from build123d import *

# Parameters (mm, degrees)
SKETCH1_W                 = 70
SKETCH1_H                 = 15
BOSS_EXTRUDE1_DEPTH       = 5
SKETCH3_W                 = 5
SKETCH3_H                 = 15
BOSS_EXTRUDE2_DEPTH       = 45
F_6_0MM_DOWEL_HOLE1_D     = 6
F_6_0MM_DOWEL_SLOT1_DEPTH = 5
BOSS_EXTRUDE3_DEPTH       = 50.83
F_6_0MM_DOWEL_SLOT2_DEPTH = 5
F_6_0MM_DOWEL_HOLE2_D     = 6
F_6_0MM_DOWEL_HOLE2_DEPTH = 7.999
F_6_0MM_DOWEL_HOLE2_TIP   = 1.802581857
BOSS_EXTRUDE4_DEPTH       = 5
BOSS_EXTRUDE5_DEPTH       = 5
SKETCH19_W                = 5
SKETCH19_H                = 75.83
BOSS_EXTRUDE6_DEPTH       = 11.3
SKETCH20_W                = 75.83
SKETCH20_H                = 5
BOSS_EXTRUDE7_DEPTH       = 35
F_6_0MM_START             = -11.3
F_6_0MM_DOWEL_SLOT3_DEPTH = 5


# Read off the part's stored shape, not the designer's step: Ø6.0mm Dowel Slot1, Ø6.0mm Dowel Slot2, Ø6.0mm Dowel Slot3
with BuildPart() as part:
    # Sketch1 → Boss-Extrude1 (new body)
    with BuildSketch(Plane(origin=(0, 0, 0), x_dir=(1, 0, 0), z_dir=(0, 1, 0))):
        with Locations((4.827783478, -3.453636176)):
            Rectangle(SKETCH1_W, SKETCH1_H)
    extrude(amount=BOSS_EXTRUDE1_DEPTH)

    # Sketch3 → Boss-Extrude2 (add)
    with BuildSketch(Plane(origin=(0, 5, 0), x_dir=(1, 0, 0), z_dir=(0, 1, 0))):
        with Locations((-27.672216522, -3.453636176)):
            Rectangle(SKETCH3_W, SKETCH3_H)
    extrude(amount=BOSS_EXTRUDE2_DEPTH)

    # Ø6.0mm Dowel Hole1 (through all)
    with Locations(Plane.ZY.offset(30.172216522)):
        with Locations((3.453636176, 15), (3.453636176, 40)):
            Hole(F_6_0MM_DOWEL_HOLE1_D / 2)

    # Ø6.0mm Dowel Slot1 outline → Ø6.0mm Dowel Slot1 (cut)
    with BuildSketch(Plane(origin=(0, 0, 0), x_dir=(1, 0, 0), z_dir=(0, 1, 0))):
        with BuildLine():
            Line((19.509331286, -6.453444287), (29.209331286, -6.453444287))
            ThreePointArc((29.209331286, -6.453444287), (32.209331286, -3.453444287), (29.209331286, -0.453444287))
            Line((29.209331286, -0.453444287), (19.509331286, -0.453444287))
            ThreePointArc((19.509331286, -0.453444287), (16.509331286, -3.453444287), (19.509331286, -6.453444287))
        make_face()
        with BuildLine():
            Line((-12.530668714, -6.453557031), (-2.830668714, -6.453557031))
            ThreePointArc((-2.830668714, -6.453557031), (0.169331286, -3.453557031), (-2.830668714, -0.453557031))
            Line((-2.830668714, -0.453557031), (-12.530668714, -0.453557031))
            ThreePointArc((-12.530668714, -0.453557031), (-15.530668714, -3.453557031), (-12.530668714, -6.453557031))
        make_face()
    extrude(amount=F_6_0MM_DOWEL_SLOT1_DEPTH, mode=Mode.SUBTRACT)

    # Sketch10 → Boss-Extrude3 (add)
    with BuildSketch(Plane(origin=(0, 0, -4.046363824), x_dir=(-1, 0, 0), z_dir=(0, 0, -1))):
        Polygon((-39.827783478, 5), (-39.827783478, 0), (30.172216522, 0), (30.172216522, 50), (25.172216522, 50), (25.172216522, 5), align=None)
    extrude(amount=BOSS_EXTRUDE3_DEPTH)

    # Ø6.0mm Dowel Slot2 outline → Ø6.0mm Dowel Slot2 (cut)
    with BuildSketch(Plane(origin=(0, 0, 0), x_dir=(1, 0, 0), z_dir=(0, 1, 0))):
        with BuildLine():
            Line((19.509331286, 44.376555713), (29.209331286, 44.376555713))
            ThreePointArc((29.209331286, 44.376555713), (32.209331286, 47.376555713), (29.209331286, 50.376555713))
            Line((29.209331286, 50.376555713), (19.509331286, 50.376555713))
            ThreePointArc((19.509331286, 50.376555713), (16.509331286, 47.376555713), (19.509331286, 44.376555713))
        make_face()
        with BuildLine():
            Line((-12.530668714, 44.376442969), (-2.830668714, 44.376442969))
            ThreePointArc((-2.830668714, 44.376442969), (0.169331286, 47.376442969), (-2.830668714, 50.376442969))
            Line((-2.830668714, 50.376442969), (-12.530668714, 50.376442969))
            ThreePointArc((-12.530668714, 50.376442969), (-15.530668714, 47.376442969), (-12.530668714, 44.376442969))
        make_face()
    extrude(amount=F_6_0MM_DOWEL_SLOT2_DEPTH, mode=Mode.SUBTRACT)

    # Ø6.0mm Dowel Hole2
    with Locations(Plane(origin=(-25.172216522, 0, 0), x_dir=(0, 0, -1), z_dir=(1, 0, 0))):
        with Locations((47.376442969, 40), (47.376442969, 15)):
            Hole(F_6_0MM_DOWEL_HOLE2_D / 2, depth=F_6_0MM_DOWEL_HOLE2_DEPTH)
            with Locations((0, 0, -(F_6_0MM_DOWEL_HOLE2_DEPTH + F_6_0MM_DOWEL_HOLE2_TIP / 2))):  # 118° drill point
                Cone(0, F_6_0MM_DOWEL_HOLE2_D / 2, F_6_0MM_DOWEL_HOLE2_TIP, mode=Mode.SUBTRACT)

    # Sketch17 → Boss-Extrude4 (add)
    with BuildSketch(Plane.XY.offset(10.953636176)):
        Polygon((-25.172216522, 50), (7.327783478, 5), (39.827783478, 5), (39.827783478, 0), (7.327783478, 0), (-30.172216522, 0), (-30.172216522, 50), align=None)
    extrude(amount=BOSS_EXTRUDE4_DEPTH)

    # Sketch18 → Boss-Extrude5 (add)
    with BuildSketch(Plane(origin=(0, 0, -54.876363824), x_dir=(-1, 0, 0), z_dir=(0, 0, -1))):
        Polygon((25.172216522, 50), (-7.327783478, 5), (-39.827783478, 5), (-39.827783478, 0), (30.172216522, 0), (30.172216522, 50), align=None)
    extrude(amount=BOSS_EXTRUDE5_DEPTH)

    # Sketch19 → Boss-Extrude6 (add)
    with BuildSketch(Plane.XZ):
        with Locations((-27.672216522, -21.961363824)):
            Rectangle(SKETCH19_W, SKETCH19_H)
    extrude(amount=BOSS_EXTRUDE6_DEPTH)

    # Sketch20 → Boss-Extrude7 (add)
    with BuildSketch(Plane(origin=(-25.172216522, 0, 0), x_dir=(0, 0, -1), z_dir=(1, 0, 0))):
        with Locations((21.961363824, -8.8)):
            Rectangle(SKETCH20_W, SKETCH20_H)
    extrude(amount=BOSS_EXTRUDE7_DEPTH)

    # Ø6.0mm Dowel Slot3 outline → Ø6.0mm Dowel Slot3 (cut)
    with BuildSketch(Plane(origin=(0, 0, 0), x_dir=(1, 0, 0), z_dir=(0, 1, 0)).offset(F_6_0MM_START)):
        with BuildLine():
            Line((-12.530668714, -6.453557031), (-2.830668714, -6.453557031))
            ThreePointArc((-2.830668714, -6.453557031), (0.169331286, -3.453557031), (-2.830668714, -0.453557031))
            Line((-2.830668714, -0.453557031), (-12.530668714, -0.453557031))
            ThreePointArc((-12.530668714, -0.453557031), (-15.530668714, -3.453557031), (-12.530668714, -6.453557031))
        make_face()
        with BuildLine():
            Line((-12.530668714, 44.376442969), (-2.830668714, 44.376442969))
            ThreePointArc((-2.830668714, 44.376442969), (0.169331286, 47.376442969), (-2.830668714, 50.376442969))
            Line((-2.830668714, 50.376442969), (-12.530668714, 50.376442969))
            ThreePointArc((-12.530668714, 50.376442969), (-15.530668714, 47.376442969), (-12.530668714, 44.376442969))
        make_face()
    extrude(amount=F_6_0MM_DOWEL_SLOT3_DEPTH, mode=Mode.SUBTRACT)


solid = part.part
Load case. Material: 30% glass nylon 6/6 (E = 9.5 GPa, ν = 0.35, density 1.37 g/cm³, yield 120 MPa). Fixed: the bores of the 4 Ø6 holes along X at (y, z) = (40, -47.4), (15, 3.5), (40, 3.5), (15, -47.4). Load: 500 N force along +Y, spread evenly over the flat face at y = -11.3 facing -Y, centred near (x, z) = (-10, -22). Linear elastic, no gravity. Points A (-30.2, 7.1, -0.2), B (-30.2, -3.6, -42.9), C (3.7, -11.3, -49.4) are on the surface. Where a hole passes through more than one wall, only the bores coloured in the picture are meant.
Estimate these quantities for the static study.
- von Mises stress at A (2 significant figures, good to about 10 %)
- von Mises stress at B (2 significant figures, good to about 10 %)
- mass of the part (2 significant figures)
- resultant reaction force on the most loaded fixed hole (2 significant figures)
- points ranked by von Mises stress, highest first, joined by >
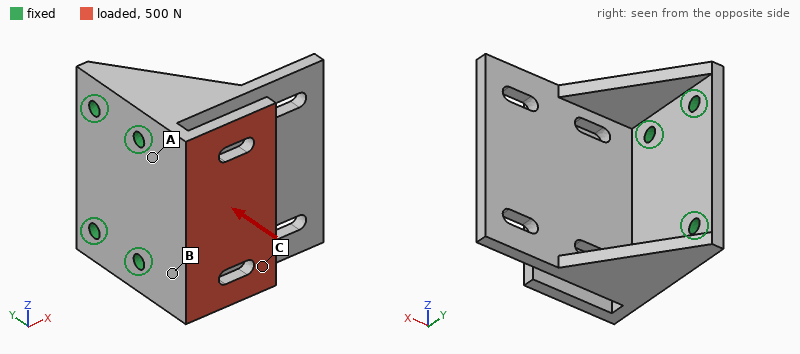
9.5 MPa
21 MPa
89 g
210 N
B > A > C
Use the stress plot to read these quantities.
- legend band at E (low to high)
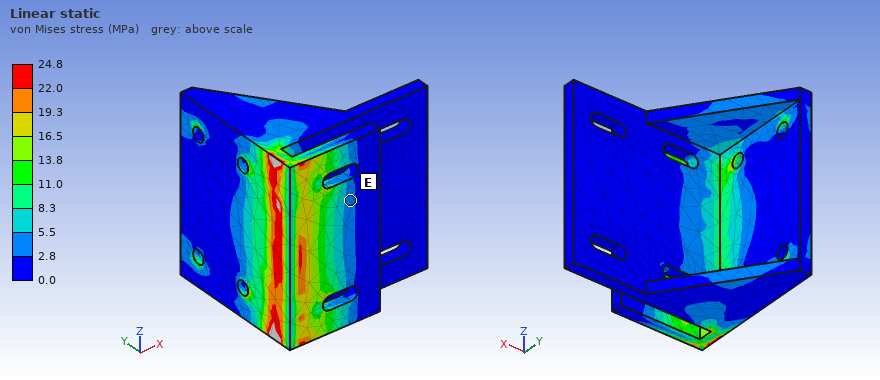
2.8 to 5.5 MPa
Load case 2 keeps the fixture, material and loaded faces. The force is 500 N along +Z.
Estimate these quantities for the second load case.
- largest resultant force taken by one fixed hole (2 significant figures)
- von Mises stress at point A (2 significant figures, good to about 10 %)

380 N
4.3 MPa
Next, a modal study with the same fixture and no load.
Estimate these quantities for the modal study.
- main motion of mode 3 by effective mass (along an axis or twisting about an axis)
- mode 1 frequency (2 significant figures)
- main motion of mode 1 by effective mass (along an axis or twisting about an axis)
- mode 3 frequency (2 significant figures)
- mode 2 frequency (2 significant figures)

along Z
790 Hz
along Y
1500 Hz
1000 Hz
